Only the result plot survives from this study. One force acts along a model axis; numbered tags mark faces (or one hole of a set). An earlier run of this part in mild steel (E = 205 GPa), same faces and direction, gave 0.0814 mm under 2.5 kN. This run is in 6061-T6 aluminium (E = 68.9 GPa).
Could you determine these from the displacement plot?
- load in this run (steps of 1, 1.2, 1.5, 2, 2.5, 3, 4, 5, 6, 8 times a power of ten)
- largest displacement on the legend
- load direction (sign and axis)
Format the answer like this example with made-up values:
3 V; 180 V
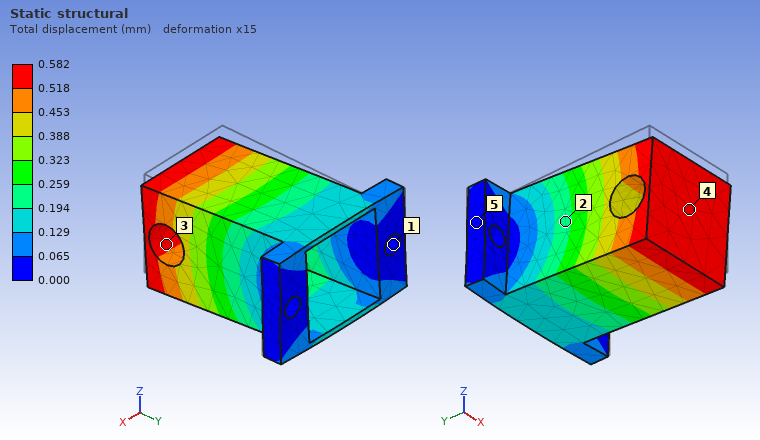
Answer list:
6 kN; 0.582 mm; -Z
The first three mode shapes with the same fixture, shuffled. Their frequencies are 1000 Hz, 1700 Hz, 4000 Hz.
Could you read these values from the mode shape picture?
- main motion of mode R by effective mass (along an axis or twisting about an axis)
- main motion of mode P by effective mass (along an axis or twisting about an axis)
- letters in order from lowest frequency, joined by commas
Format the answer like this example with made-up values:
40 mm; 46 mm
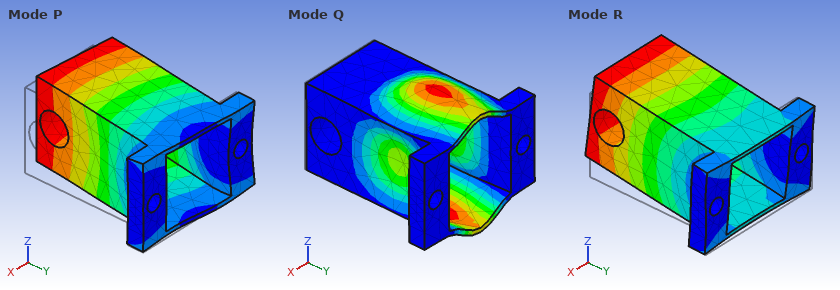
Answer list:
along Z; along X; R, P, Q
